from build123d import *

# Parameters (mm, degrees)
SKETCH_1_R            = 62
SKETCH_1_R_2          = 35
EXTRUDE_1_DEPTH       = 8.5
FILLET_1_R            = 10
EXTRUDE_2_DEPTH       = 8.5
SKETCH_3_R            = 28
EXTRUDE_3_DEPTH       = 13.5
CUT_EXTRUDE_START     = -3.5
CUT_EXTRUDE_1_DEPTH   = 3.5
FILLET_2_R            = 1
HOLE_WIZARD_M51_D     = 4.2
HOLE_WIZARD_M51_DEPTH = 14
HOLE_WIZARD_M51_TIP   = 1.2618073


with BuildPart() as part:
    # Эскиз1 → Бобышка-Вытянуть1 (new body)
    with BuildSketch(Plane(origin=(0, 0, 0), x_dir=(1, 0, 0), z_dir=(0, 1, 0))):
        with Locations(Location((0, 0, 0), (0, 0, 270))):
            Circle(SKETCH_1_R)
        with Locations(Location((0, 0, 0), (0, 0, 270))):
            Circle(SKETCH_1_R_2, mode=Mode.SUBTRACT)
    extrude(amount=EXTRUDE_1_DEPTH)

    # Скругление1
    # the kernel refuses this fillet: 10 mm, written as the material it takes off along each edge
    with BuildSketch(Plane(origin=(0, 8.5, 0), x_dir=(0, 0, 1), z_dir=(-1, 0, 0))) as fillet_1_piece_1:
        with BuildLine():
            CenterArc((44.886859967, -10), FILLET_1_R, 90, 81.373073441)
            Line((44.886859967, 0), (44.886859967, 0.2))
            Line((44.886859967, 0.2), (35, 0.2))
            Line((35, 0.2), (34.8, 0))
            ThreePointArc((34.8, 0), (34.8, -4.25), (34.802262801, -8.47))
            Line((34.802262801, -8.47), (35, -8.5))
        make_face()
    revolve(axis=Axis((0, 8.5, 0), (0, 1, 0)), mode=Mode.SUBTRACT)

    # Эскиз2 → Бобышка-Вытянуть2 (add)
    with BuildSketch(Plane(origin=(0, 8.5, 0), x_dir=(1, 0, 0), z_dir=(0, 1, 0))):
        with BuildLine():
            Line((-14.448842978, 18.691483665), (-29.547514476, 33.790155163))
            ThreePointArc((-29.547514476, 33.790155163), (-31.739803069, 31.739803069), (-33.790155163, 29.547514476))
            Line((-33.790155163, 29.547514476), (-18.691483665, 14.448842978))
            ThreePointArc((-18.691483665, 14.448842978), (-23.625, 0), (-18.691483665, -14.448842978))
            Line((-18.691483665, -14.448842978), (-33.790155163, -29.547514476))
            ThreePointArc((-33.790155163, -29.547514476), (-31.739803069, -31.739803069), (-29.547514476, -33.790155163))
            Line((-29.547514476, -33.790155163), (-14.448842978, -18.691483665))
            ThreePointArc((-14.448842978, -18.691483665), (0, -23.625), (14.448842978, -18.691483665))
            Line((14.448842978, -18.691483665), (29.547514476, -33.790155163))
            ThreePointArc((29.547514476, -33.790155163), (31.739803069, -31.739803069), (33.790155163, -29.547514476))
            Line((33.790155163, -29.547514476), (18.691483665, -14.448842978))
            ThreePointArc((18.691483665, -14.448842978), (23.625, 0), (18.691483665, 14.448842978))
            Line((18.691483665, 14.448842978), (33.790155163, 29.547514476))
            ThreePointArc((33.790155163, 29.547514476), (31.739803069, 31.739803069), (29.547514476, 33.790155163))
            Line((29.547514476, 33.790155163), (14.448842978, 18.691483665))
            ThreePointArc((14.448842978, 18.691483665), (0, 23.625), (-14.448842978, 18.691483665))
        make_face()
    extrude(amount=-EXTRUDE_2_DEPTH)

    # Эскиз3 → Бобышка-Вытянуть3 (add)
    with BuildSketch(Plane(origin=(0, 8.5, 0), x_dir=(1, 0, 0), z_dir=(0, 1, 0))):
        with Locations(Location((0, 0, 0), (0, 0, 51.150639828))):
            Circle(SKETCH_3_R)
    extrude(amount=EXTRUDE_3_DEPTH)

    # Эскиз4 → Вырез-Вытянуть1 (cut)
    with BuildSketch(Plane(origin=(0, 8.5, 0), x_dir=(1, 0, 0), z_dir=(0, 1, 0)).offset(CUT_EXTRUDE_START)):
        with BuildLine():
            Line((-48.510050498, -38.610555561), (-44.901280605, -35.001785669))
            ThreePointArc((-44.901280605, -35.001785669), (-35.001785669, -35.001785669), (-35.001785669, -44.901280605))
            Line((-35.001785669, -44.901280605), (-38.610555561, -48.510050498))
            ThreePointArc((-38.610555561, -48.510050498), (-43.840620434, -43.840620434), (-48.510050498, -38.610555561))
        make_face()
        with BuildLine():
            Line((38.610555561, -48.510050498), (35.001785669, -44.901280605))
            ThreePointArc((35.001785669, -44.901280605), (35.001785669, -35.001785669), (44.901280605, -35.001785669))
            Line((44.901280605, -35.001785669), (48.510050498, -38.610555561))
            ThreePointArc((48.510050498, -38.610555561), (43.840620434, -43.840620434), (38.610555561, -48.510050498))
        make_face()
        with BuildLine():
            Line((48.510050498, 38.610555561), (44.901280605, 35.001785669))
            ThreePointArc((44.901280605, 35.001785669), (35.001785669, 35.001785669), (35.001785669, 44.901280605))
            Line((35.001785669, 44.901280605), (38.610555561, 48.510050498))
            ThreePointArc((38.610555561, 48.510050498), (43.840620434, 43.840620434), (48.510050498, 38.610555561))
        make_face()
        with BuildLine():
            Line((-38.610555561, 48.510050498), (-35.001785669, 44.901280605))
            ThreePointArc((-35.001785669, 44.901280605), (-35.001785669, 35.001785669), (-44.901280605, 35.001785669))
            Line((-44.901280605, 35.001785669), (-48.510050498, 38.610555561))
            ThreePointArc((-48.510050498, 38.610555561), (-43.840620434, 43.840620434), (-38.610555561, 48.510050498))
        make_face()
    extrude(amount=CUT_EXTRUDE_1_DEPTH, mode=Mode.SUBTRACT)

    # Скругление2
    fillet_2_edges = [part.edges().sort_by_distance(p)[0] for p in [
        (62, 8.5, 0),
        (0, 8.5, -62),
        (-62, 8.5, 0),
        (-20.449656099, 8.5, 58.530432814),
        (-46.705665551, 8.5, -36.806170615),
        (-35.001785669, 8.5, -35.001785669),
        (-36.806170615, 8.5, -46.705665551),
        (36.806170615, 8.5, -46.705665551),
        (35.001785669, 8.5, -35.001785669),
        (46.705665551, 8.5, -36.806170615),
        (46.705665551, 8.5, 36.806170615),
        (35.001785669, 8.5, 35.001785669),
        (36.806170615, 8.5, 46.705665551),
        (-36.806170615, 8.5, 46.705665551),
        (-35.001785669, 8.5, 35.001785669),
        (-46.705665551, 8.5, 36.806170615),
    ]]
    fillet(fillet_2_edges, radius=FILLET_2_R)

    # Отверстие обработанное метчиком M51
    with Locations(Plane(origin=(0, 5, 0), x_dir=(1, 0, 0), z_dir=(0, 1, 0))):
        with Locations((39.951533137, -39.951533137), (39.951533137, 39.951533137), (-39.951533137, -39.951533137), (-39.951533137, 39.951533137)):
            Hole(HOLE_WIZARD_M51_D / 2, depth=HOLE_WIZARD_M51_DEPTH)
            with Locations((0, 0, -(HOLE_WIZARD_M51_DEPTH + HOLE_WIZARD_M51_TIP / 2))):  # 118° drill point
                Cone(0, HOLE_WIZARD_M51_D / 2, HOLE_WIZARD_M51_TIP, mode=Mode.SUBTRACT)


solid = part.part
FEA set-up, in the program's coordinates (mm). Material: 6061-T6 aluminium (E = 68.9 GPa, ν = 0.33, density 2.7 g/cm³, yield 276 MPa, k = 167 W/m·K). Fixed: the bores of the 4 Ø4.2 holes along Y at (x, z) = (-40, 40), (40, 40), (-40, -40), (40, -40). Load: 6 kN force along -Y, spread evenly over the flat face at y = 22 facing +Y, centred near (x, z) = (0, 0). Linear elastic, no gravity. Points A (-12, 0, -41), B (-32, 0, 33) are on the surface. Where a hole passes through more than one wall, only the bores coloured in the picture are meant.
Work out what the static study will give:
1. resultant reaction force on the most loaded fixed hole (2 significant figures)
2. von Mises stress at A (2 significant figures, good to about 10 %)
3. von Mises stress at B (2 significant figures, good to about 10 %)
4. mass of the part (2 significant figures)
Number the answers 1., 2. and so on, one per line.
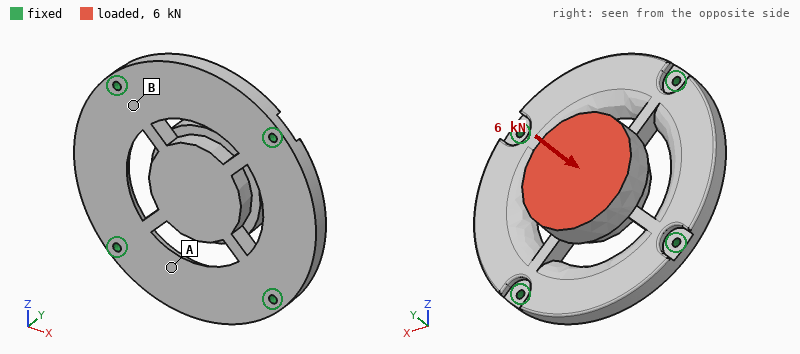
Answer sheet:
1. 2.5 kN
2. 22 MPa
3. 53 MPa
4. 310 g
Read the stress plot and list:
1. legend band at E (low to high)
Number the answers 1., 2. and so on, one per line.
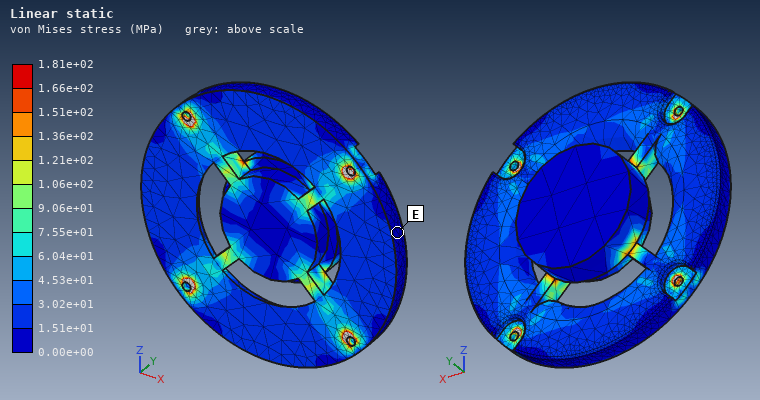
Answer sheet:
1. 0.00e+00 to 1.51e+01 MPa
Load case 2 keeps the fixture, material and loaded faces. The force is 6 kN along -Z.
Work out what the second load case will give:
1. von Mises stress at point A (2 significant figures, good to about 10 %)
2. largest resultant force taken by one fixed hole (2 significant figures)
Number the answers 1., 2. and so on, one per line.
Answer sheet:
1. 12 MPa
2. 2.0 kN
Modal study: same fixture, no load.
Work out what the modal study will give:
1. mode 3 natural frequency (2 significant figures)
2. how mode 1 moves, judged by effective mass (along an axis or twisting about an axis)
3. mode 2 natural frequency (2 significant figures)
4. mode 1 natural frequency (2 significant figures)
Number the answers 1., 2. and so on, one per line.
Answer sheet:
1. 4100 Hz
2. along Y
3. 3600 Hz
4. 2600 Hz
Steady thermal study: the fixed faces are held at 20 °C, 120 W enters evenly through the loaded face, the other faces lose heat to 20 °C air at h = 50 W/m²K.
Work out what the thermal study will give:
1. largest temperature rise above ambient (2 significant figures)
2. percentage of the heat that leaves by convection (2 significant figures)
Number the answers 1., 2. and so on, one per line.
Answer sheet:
1. 66 K
2. 25 %
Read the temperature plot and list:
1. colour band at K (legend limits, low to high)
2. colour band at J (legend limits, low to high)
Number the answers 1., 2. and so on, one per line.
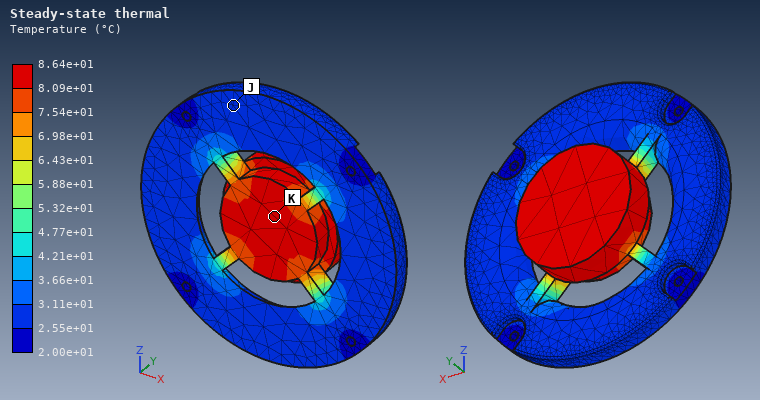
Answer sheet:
1. 8.09e+01 to 8.64e+01 °C
2. 2.55e+01 to 3.11e+01 °C
